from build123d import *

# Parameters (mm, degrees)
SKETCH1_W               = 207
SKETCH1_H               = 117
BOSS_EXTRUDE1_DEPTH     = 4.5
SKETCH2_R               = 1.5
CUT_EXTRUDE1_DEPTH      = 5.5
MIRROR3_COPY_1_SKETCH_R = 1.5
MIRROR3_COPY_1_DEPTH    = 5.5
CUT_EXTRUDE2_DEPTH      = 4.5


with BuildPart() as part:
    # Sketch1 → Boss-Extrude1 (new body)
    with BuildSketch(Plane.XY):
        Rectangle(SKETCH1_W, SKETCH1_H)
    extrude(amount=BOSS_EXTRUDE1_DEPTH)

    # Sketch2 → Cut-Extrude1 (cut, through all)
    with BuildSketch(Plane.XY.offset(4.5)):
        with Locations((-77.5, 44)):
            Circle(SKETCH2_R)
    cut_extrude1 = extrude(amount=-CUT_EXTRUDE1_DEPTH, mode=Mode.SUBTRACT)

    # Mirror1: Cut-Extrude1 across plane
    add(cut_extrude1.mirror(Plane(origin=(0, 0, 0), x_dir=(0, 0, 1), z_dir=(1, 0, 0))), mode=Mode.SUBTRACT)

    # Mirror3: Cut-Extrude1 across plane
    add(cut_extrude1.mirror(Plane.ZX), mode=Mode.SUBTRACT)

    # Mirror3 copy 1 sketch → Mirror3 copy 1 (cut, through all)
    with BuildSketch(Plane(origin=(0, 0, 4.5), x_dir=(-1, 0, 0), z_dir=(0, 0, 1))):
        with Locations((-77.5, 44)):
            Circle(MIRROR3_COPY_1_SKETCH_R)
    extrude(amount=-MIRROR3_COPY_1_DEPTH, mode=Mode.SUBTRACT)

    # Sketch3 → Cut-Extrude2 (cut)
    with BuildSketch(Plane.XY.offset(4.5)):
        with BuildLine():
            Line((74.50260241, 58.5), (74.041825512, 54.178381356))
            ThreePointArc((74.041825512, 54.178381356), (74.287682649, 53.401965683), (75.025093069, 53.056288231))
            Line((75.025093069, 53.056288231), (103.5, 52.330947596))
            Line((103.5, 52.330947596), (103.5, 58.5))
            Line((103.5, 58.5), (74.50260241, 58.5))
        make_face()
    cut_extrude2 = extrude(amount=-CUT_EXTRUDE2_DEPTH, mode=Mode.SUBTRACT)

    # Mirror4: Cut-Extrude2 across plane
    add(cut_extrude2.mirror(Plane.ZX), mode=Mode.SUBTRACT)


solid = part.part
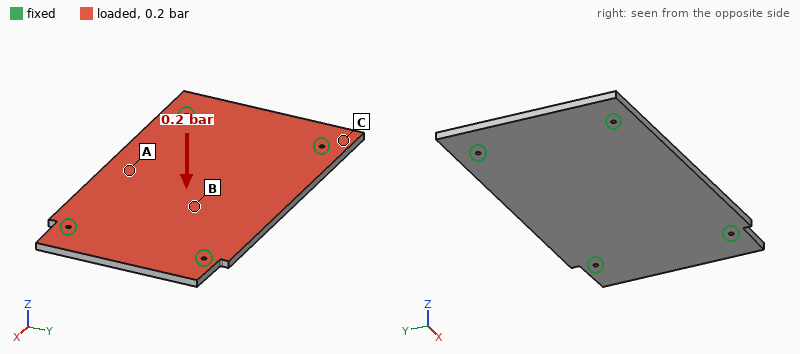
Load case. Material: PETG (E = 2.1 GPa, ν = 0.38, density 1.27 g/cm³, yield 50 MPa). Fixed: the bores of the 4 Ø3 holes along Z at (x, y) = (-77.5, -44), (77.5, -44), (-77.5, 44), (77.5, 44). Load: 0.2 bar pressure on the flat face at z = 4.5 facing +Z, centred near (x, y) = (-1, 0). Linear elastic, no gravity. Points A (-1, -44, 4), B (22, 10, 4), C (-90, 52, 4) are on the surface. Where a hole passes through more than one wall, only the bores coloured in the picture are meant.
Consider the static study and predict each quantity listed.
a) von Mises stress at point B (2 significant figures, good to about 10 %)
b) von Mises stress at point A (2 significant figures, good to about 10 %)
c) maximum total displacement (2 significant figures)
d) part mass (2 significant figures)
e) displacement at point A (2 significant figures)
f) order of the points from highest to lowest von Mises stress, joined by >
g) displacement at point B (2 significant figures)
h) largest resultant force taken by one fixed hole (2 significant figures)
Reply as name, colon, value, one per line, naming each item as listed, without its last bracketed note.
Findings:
von Mises stress at point B: 5.1 MPa
von Mises stress at point A: 7.0 MPa
maximum total displacement: 2.7 mm
part mass: 140 g
displacement at point A: 2.7 mm
order of the points from highest to lowest von Mises stress, joined by >: A > B > C
displacement at point B: 2.4 mm
largest resultant force taken by one fixed hole: 120 N
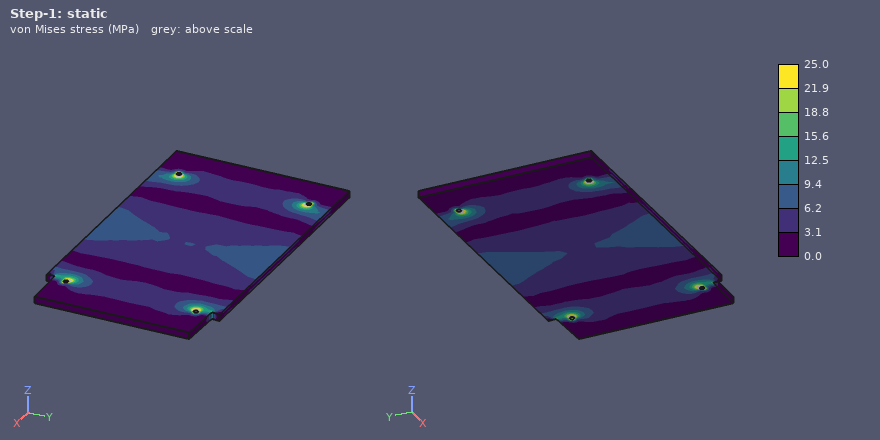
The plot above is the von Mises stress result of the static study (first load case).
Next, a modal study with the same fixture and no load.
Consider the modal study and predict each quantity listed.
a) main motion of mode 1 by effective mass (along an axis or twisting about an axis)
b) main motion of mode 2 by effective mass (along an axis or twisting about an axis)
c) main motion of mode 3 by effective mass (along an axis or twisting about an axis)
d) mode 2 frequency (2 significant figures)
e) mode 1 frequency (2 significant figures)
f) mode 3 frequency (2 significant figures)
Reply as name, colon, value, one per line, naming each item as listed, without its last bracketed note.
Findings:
main motion of mode 1 by effective mass: along Z
main motion of mode 2 by effective mass: twisting about X
main motion of mode 3 by effective mass: twisting about Y
mode 2 frequency: 310 Hz
mode 1 frequency: 200 Hz
mode 3 frequency: 540 Hz
